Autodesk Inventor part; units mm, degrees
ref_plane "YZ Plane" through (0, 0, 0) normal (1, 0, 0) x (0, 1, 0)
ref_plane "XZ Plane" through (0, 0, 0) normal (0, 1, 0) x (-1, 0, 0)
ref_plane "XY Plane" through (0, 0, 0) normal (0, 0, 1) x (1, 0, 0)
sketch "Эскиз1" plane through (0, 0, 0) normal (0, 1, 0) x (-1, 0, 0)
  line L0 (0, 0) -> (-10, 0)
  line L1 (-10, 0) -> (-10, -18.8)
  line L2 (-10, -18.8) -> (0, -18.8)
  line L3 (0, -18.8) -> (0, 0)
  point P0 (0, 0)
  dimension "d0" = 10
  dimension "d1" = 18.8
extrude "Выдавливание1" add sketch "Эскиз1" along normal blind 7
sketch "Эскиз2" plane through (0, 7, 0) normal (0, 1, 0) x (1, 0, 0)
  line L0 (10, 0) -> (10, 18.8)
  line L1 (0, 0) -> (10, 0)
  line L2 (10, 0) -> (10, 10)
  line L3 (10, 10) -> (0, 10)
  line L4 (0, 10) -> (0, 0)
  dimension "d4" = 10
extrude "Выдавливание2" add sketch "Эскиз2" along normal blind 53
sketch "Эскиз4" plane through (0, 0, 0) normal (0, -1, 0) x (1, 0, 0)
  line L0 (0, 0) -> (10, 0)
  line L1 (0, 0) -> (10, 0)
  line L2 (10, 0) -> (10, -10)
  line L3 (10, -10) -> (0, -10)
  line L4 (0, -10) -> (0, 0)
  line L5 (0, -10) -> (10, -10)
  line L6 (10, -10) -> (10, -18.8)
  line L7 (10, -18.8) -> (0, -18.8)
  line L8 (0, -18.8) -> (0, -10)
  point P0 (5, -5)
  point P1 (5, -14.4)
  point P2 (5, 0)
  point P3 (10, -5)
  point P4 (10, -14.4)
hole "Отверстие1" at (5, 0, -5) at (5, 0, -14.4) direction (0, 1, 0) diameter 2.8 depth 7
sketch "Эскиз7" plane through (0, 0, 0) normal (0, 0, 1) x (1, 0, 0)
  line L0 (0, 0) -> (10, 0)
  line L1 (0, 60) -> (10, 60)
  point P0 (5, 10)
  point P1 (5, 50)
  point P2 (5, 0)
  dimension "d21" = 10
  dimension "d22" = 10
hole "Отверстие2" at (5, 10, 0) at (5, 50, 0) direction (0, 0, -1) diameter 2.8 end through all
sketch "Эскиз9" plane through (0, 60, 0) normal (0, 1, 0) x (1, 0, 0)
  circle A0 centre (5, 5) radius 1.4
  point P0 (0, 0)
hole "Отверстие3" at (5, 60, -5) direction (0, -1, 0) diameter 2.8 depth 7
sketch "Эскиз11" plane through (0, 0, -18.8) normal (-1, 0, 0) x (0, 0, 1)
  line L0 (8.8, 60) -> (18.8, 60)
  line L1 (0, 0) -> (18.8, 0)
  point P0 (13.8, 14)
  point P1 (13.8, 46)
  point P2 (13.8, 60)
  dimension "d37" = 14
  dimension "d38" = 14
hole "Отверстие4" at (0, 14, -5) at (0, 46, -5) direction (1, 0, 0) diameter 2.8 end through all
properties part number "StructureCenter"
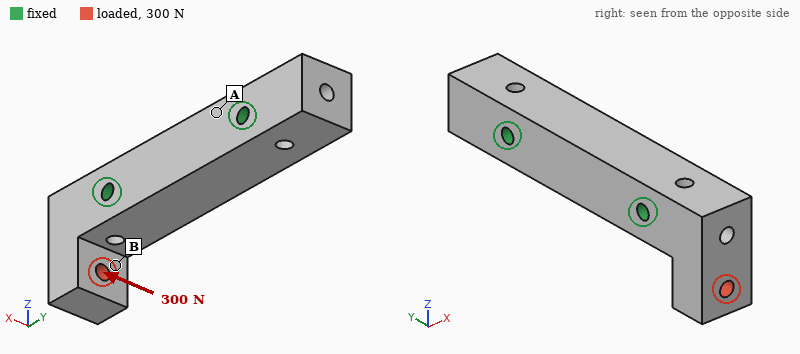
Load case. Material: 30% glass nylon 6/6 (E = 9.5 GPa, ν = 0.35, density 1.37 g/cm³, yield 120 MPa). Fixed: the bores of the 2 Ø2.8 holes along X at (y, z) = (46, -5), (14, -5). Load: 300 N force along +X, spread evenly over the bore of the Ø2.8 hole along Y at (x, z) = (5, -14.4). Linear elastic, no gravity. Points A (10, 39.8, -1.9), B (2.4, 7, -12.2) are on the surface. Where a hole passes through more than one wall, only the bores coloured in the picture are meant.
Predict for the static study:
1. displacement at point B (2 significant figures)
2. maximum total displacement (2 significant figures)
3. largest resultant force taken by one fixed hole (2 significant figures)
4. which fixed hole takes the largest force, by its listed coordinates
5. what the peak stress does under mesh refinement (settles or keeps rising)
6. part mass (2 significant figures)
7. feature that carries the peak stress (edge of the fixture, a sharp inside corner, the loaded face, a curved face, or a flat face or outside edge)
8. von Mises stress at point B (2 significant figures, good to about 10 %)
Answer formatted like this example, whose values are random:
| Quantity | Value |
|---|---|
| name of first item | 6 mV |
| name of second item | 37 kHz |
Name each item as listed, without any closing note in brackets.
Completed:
| Quantity | Value |
|---|---|
| displacement at point B | 0.068 mm |
| maximum total displacement | 0.14 mm |
| largest resultant force taken by one fixed hole | 310 N |
| which fixed hole takes the largest force, by its listed coordinates | (14, -5) |
| what the peak stress does under mesh refinement | keeps rising |
| part mass | 8.5 g |
| feature that carries the peak stress | edge of the fixture |
| von Mises stress at point B | 11 MPa |
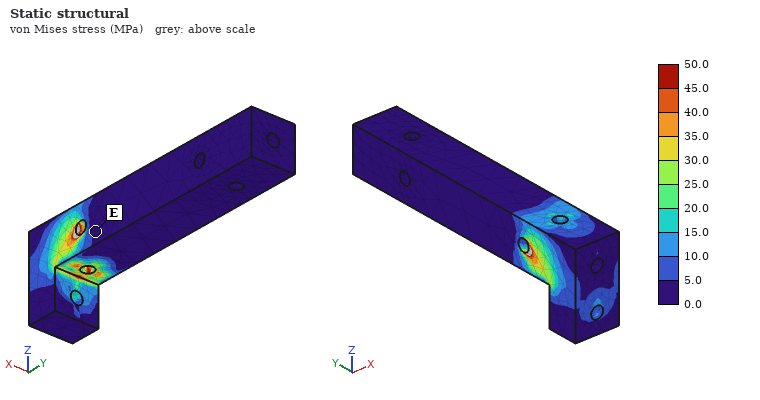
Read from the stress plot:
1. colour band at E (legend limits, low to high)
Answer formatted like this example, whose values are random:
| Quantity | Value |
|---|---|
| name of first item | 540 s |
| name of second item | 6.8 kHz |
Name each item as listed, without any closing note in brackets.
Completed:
| Quantity | Value |
|---|---|
| colour band at E | 0.0 to 5.0 MPa |
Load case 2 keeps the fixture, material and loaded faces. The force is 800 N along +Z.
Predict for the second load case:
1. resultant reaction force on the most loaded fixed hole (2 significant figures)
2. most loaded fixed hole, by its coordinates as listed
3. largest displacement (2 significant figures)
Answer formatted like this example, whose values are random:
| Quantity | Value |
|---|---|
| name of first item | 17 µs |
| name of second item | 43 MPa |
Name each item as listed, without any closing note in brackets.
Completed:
| Quantity | Value |
|---|---|
| resultant reaction force on the most loaded fixed hole | 930 N |
| most loaded fixed hole, by its coordinates as listed | (14, -5) |
| largest displacement | 0.25 mm |
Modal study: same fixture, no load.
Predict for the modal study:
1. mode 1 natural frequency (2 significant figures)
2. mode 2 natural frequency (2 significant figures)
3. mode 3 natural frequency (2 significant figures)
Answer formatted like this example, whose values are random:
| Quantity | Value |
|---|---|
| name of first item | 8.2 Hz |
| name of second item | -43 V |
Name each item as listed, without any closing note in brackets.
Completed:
| Quantity | Value |
|---|---|
| mode 1 natural frequency | 7400 Hz |
| mode 2 natural frequency | 8900 Hz |
| mode 3 natural frequency | 12 kHz |
